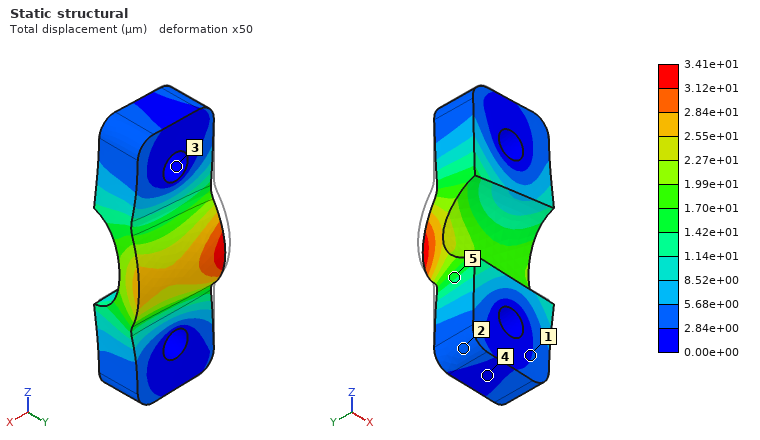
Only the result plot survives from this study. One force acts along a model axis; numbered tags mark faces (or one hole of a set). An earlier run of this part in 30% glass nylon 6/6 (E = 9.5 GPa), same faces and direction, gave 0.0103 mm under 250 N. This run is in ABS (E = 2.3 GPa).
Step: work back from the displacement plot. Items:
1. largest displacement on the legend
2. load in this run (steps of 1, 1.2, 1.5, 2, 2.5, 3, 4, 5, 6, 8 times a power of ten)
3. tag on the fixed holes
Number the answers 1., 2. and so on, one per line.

1. 3.41e+01 µm
2. 200 N
3. 3
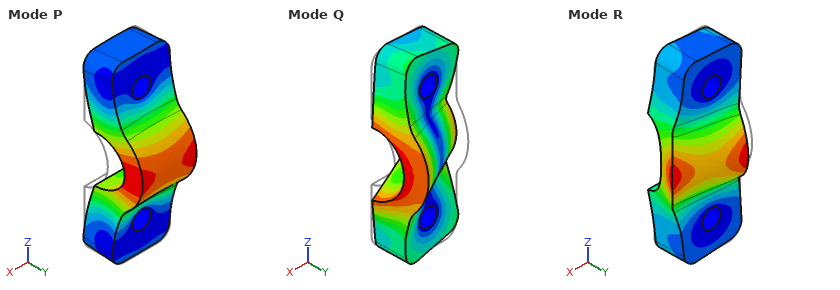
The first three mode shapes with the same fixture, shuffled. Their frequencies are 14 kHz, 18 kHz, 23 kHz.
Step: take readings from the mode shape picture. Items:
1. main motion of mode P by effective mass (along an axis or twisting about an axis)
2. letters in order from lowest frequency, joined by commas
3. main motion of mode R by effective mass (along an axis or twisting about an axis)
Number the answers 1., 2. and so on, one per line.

1. along Y
2. R, P, Q
3. along X
